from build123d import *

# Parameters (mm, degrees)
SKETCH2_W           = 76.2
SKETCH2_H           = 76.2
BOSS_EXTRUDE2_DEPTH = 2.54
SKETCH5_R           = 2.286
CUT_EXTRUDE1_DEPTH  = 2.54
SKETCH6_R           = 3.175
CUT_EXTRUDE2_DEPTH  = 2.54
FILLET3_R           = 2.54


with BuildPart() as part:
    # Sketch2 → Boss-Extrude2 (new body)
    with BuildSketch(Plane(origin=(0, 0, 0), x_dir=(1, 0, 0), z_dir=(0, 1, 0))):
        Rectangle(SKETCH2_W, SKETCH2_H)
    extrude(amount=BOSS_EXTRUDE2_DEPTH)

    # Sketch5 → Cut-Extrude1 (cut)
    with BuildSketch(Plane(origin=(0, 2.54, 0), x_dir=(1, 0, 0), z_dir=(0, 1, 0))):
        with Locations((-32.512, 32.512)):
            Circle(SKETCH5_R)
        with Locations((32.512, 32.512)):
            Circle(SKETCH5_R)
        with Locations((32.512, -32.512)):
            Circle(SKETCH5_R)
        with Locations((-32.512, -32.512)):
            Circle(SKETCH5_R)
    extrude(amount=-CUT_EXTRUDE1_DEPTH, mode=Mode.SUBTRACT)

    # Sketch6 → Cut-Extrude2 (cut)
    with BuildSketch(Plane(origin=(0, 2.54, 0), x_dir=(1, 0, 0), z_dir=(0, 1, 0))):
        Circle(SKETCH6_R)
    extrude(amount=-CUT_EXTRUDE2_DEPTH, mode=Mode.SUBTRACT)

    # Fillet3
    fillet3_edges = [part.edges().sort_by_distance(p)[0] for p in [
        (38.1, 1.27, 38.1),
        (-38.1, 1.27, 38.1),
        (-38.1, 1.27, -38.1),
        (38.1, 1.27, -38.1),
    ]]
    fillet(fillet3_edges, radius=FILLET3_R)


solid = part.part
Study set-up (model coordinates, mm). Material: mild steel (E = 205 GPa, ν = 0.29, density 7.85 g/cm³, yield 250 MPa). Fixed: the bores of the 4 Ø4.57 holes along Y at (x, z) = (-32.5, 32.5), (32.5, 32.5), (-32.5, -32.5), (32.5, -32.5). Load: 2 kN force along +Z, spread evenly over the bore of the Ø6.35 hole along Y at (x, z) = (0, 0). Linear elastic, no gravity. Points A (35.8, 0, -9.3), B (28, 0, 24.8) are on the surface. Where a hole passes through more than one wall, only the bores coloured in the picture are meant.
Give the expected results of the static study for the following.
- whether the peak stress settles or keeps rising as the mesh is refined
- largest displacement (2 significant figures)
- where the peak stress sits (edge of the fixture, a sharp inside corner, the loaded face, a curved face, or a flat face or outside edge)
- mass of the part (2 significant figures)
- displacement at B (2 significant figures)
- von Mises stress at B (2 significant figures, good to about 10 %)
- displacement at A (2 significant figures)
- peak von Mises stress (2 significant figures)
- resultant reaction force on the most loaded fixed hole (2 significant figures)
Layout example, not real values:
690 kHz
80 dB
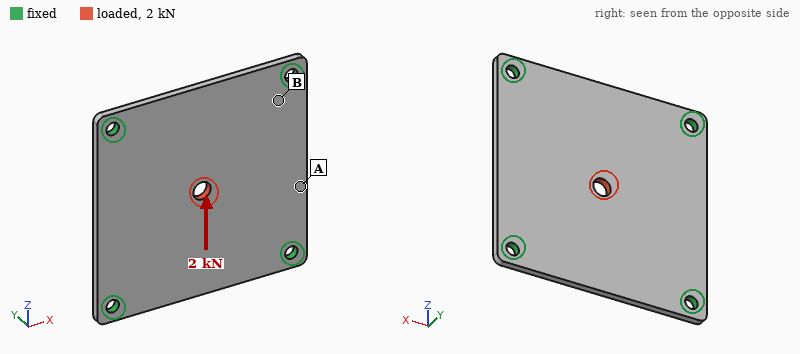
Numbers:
settles
4.1 µm
the loaded face
110 g
0.71 µm
15 MPa
0.85 µm
70 MPa
570 N
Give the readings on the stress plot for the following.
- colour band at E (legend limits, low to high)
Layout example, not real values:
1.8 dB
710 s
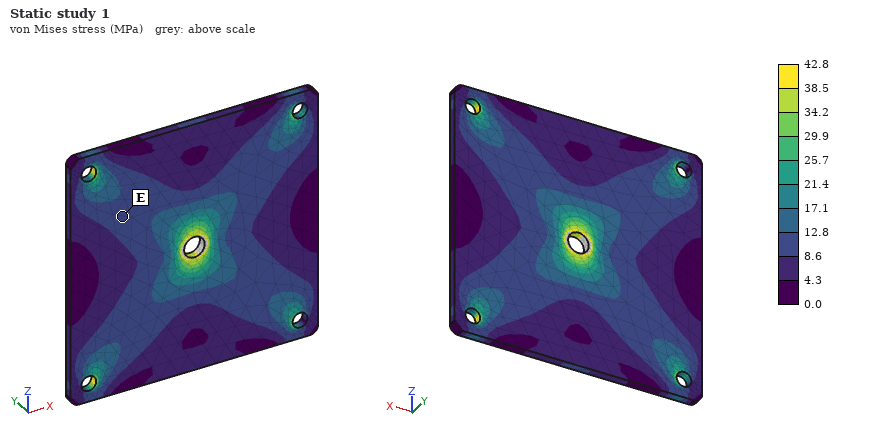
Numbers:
8.6 to 12.8 MPa
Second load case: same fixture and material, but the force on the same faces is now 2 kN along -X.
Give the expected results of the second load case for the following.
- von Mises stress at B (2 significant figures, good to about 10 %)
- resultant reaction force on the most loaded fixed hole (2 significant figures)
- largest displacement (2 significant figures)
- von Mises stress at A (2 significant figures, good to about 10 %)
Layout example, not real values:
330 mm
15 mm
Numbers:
14 MPa
570 N
4.1 µm
5.4 MPa
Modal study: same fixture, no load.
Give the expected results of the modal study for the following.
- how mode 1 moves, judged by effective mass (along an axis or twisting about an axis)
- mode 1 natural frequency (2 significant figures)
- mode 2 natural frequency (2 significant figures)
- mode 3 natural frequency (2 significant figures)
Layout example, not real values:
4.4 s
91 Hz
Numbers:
along Y
2100 Hz
3600 Hz
3600 Hz
